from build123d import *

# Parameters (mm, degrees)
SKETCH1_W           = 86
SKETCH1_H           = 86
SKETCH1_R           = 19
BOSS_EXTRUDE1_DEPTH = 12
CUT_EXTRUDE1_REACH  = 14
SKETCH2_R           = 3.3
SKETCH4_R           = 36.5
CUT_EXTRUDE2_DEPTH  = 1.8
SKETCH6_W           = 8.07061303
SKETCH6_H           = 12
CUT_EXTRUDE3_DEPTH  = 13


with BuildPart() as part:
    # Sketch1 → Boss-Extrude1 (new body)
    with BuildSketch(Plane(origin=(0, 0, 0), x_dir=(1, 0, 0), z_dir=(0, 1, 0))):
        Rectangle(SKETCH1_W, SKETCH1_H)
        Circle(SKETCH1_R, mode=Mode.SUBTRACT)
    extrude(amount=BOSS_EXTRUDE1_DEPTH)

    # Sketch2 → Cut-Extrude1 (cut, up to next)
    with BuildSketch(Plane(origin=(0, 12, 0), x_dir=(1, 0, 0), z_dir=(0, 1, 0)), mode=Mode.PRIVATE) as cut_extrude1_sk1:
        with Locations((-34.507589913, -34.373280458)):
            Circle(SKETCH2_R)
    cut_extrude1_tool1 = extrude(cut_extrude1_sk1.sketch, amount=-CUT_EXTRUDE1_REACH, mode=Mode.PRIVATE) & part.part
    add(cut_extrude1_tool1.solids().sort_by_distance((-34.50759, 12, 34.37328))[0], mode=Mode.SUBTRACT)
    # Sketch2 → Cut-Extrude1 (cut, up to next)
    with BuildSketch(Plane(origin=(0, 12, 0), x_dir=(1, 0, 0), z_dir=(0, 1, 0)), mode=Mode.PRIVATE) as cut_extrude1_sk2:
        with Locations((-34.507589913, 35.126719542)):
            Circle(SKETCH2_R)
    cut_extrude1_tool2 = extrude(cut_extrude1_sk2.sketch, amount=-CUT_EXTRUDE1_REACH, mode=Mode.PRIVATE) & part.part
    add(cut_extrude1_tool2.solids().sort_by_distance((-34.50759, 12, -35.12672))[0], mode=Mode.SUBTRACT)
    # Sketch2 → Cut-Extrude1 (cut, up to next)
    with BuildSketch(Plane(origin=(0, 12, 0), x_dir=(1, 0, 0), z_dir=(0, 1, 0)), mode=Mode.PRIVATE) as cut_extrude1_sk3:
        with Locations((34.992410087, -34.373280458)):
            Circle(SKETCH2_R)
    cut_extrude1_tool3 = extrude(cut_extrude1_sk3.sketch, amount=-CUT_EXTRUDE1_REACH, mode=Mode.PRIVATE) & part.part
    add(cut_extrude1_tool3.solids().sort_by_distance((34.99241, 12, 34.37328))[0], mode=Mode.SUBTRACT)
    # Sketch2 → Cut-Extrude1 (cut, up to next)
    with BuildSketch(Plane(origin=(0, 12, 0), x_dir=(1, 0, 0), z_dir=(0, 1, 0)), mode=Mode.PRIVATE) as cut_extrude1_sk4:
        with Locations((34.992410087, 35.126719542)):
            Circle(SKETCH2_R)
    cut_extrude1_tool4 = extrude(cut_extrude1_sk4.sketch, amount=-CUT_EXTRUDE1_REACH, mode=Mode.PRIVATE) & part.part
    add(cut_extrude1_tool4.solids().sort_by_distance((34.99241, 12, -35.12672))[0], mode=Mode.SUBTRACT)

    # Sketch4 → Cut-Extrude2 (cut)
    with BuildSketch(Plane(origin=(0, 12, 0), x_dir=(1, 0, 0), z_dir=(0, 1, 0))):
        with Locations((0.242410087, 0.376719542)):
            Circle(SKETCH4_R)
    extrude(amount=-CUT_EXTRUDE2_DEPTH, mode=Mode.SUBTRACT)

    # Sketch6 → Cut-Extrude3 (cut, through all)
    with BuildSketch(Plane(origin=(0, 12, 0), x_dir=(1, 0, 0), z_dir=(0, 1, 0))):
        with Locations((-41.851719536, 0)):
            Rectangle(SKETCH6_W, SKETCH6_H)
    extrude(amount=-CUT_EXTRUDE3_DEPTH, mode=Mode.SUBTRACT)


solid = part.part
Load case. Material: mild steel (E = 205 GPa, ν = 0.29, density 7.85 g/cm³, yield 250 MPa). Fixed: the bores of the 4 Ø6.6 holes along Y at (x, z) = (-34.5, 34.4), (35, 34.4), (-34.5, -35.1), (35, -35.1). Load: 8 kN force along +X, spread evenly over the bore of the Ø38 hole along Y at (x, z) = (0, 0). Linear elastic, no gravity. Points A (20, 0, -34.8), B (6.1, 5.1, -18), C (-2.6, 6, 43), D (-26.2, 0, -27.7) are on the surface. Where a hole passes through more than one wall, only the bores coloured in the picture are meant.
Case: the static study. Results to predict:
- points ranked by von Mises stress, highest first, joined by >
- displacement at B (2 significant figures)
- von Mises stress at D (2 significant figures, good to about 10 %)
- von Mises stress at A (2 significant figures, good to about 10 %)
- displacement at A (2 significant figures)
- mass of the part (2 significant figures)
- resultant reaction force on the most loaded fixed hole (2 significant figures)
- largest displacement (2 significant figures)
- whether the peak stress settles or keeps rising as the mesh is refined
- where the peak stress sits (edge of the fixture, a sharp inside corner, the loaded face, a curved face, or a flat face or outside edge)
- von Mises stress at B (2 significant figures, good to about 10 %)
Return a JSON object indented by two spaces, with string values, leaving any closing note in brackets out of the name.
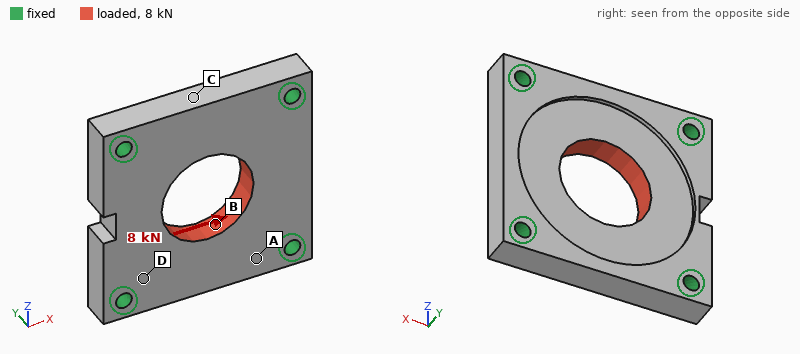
{
  "points ranked by von Mises stress, highest first, joined by >": "B > D > A > C",
  "displacement at B": "1.5 µm",
  "von Mises stress at D": "9.9 MPa",
  "von Mises stress at A": "6.4 MPa",
  "displacement at A": "0.51 µm",
  "mass of the part": "530 g",
  "resultant reaction force on the most loaded fixed hole": "2.2 kN",
  "largest displacement": "2.7 µm",
  "whether the peak stress settles or keeps rising as the mesh is refined": "keeps rising",
  "where the peak stress sits": "edge of the fixture",
  "von Mises stress at B": "13 MPa"
}
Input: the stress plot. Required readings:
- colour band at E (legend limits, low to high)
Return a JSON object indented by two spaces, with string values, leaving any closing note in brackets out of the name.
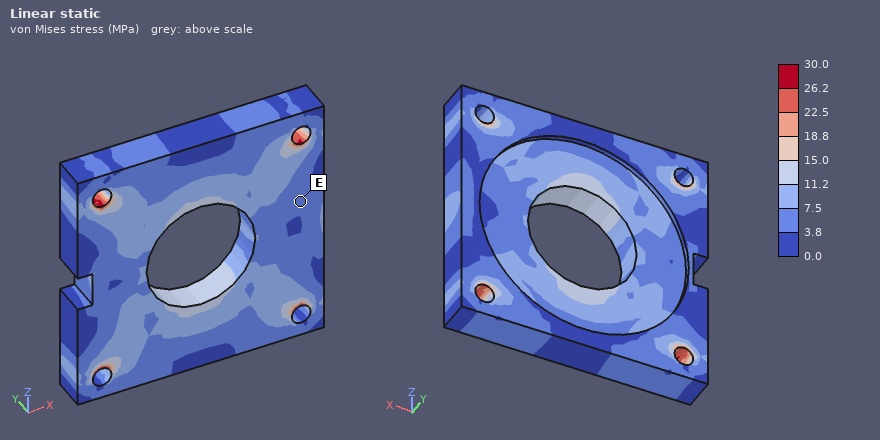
{
  "colour band at E": "3.8 to 7.5 MPa"
}
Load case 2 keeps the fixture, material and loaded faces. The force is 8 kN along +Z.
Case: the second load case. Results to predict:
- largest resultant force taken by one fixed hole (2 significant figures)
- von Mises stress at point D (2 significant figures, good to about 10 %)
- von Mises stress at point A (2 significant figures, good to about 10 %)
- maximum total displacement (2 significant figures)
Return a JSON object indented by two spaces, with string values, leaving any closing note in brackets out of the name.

{
  "largest resultant force taken by one fixed hole": "2.2 kN",
  "von Mises stress at point D": "10 MPa",
  "von Mises stress at point A": "6.4 MPa",
  "maximum total displacement": "2.5 µm"
}
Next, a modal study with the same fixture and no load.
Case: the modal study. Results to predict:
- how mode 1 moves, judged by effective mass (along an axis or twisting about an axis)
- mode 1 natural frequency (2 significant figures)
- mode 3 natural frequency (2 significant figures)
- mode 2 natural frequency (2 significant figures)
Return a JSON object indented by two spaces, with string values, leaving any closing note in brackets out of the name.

{
  "how mode 1 moves, judged by effective mass": "along Y",
  "mode 1 natural frequency": "8900 Hz",
  "mode 3 natural frequency": "12 kHz",
  "mode 2 natural frequency": "11 kHz"
}
